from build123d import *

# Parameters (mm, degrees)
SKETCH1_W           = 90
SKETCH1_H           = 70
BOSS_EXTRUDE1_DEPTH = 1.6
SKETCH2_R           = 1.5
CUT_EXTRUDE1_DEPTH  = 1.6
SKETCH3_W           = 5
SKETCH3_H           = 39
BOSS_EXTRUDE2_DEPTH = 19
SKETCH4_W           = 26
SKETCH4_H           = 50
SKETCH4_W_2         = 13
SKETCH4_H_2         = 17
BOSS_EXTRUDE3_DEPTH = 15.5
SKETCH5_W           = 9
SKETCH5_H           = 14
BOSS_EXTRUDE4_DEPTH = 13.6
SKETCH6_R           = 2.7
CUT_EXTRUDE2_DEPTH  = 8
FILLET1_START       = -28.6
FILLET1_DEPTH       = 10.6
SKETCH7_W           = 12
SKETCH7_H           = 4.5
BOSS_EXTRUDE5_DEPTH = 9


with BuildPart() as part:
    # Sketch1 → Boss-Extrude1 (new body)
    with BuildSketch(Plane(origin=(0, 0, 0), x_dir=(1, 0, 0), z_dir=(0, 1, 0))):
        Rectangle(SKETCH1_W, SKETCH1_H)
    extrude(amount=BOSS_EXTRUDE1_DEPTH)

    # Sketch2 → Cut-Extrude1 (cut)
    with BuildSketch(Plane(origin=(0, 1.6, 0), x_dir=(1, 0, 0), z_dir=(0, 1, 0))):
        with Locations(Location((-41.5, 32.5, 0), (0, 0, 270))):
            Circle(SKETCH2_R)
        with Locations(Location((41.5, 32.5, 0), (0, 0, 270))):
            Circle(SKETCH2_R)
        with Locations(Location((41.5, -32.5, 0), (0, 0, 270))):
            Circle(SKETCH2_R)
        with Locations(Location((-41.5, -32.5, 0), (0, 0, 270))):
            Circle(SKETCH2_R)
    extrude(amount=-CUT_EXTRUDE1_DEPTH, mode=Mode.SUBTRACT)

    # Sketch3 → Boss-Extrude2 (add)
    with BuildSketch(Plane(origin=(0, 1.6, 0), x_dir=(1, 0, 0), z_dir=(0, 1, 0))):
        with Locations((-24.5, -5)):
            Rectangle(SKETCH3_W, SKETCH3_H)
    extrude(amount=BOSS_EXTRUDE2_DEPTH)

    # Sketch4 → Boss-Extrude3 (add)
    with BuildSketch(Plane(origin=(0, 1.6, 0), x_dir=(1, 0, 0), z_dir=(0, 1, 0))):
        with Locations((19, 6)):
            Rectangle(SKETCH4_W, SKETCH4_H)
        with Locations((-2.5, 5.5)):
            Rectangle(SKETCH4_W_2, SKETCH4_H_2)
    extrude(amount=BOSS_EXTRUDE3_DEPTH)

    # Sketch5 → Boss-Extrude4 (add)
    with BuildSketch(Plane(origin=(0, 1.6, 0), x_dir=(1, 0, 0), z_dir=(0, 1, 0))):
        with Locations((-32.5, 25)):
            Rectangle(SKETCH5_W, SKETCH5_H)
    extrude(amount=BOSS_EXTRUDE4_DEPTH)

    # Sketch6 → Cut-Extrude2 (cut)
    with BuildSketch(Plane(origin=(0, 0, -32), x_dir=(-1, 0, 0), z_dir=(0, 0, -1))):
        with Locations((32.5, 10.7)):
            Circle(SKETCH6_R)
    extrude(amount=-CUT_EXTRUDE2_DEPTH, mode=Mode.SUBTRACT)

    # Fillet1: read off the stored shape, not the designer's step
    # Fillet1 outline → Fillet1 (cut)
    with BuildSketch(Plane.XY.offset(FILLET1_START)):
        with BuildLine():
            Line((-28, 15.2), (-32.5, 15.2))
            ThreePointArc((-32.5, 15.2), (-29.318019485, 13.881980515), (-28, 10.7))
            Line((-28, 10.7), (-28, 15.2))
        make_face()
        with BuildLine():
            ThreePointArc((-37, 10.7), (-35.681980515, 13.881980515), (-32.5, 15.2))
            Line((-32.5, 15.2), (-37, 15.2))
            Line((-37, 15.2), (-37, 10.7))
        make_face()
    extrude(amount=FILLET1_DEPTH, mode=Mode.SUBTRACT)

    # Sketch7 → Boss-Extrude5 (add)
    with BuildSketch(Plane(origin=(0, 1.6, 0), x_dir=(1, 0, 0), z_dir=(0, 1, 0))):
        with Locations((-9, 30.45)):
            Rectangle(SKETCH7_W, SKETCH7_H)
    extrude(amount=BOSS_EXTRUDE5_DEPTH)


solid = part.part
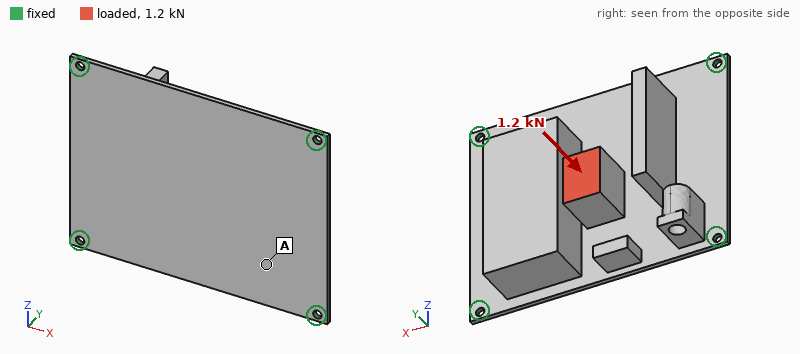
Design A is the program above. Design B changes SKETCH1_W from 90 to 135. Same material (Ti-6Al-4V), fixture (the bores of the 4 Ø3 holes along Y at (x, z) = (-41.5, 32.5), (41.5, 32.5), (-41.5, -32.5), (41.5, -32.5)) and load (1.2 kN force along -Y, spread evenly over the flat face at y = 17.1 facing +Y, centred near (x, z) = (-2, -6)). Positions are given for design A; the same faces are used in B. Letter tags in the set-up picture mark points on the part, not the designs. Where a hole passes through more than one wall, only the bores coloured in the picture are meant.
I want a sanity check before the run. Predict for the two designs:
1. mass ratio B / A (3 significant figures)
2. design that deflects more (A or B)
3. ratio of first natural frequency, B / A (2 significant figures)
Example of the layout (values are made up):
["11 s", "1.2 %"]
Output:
["1.13", "A", "1.0"]
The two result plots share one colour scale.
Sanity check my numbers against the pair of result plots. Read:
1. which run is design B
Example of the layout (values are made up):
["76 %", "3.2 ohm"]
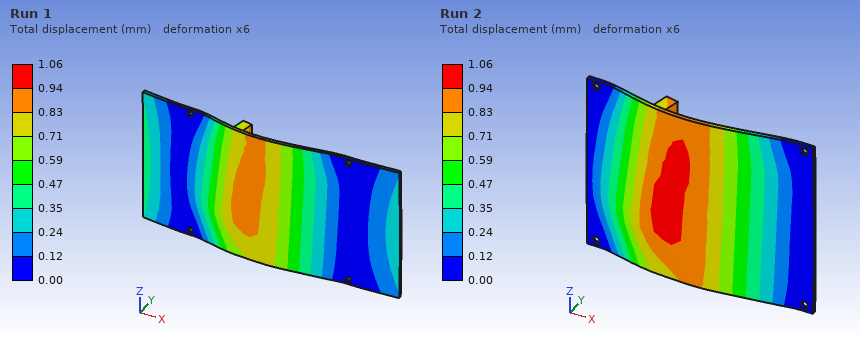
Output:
["Run 1"]
